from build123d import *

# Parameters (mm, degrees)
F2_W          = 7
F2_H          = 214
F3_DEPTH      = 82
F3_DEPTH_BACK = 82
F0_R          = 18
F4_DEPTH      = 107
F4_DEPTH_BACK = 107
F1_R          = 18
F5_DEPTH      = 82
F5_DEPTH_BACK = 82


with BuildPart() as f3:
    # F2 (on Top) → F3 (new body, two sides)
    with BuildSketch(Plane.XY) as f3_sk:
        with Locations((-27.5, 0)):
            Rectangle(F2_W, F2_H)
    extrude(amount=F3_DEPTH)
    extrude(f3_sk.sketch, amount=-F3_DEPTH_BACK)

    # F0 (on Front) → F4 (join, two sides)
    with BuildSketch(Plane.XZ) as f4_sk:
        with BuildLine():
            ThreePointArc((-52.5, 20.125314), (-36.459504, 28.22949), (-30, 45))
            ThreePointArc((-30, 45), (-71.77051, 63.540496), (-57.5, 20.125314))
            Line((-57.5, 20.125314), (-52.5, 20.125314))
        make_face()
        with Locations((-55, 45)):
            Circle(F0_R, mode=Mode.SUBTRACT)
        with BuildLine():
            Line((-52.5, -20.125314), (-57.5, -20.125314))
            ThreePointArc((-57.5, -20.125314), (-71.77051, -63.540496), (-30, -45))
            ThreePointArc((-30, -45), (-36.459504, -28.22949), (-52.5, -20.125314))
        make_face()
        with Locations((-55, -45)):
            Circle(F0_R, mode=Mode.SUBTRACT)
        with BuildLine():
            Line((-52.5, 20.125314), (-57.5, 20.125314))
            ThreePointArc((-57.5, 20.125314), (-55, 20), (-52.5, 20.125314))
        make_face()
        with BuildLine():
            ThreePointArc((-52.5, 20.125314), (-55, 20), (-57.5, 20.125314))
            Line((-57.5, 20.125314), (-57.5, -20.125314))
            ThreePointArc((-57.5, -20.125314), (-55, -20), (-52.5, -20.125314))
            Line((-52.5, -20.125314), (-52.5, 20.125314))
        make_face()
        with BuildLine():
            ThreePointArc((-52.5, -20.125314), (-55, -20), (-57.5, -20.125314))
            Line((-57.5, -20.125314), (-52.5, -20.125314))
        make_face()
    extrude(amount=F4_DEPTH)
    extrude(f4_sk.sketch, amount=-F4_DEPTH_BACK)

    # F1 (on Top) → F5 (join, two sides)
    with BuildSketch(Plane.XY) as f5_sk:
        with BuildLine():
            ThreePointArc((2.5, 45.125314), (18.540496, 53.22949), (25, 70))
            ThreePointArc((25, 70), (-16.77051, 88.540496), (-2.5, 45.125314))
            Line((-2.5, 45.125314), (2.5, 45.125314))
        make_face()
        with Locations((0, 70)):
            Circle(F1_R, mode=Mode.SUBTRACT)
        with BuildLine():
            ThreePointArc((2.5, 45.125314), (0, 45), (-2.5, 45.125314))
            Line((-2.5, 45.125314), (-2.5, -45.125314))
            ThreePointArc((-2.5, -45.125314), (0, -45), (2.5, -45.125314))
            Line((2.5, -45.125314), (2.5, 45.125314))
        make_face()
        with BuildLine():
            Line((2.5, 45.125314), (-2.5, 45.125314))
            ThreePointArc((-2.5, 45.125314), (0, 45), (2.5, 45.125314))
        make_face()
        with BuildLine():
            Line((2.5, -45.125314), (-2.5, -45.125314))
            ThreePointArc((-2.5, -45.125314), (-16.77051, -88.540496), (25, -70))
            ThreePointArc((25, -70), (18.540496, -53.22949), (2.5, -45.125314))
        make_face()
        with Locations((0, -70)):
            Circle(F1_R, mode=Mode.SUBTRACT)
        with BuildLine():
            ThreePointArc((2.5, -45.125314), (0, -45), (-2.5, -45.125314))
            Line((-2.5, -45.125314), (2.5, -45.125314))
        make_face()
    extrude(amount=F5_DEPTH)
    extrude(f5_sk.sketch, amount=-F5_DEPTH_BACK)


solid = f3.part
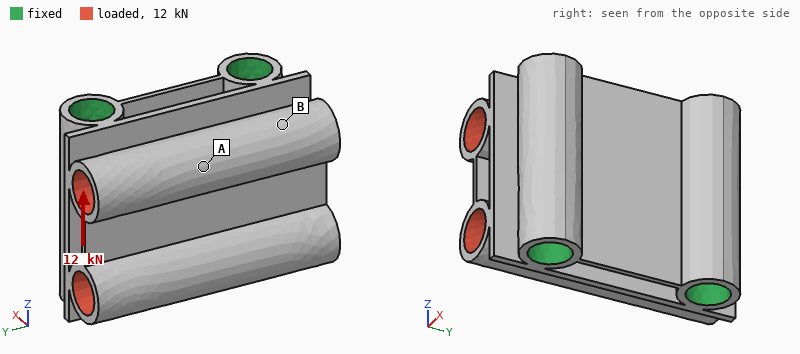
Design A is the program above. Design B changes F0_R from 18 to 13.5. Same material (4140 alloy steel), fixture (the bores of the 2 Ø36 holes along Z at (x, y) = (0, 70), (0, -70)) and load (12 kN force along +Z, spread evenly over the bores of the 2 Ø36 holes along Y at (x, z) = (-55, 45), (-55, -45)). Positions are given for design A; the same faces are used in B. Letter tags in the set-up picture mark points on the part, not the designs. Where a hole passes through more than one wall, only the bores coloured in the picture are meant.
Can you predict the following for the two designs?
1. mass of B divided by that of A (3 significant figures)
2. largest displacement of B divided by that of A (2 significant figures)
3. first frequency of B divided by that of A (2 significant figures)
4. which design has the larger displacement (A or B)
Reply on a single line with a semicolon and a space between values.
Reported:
1.18; 0.73; 1.0; A
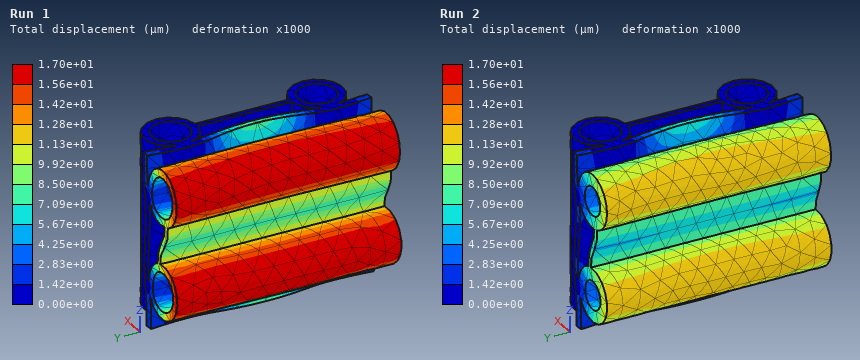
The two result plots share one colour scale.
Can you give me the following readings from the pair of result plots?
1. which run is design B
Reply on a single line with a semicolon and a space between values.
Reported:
Run 2
